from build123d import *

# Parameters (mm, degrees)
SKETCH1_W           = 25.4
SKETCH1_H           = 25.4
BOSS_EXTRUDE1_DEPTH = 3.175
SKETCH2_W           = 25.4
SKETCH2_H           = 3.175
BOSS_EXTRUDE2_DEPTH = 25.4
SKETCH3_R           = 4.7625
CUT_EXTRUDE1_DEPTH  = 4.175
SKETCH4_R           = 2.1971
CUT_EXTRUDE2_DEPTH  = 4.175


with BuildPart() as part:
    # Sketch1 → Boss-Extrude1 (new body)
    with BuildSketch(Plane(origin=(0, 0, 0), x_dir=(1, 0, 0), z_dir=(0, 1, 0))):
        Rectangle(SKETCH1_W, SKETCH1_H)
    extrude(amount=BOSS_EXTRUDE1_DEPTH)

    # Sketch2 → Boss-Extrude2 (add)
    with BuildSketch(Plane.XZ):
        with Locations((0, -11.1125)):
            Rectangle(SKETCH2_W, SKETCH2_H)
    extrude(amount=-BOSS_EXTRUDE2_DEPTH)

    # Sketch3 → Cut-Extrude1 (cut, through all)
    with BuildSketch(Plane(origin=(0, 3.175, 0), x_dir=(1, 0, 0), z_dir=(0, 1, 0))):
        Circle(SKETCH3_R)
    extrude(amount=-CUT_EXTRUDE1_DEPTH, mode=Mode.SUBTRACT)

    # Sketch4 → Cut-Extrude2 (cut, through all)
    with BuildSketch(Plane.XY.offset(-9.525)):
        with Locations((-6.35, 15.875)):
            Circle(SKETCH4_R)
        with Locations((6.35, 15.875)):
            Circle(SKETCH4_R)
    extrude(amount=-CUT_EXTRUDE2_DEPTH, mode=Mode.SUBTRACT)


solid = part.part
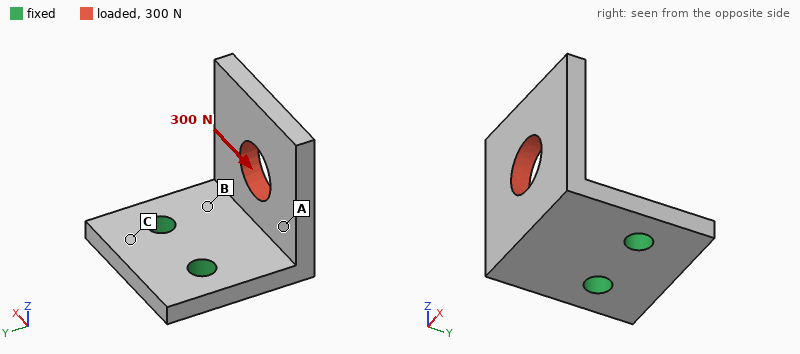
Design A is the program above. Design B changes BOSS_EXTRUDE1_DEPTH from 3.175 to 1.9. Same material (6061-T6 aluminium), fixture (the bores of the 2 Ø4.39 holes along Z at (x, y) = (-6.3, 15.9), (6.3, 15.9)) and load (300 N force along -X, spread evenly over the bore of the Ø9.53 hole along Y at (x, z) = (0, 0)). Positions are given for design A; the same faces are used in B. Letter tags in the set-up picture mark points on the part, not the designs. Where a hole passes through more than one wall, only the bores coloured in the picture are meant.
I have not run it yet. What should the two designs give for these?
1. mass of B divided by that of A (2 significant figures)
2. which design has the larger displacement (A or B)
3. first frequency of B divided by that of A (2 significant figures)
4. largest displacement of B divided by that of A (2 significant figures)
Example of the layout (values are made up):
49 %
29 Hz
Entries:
0.82
B
0.90
1.4
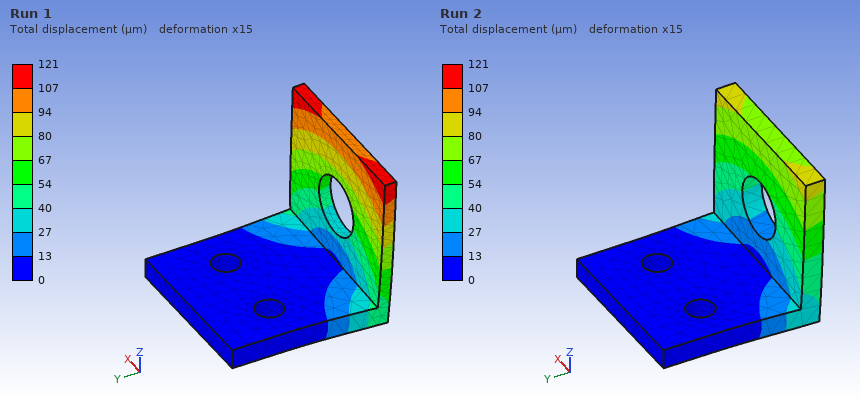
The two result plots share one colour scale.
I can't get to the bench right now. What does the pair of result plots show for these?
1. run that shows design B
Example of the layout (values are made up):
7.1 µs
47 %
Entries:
Run 1
